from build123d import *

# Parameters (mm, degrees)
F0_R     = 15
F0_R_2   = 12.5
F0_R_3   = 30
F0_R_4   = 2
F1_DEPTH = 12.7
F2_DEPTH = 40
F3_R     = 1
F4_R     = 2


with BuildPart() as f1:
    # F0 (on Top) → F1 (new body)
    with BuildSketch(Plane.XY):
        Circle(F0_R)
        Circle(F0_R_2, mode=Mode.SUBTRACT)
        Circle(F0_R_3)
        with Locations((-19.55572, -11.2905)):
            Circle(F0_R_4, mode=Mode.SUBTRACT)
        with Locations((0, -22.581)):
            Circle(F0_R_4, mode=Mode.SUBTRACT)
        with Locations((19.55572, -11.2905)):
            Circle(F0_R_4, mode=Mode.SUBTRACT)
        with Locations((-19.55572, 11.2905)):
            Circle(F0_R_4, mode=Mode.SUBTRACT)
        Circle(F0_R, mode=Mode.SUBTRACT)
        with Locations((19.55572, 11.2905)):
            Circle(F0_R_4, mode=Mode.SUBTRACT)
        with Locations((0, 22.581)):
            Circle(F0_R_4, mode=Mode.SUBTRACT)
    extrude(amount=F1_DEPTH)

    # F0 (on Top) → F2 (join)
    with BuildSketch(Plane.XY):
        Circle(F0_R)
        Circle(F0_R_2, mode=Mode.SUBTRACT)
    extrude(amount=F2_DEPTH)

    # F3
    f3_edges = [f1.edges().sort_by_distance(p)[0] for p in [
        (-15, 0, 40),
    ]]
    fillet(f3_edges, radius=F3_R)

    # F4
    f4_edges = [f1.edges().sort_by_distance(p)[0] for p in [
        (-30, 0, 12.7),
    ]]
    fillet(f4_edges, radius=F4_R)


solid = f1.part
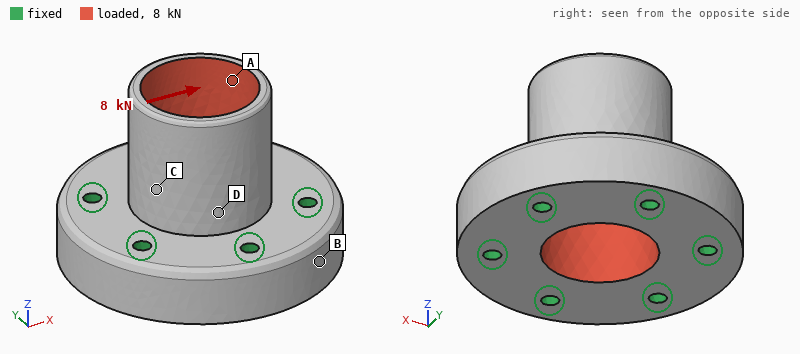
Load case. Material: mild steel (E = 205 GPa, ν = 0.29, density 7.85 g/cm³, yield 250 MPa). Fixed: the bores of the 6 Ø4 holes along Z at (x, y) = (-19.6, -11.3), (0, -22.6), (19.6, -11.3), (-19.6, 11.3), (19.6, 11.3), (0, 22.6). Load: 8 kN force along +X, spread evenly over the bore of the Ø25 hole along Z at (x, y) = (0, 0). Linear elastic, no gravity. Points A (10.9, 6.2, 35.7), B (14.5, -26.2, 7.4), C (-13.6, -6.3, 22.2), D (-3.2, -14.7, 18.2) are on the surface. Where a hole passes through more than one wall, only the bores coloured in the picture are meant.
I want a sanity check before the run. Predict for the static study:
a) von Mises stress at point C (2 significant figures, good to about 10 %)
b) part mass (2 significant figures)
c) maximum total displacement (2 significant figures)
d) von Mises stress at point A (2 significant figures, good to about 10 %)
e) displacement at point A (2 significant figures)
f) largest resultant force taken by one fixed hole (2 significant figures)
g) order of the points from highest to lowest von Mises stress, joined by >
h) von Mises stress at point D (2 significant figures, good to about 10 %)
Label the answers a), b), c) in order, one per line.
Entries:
a) 28 MPa
b) 270 g
c) 17 µm
d) 16 MPa
e) 15 µm
f) 2.2 kN
g) D > C > A > B
h) 53 MPa
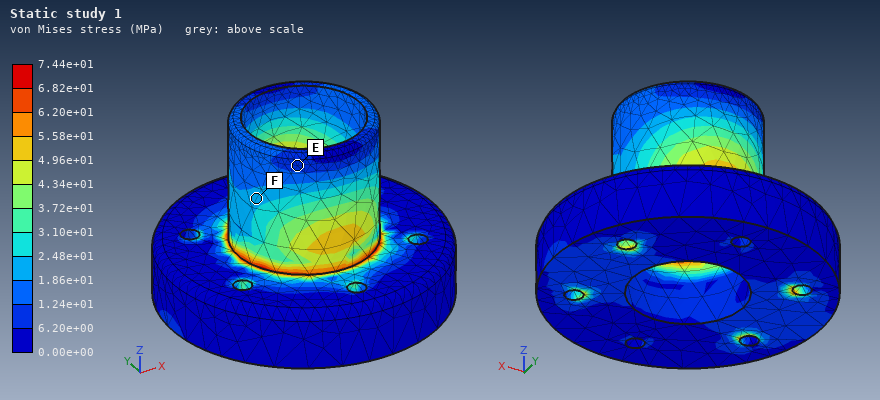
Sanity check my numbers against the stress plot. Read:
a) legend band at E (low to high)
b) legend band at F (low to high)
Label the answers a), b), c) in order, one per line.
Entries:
a) 6.20e+00 to 1.24e+01 MPa
b) 1.86e+01 to 2.48e+01 MPa
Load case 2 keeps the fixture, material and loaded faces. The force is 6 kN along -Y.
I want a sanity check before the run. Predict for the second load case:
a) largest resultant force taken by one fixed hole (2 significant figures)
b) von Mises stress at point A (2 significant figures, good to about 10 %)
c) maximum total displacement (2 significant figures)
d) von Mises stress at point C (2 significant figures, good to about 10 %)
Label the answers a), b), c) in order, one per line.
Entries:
a) 1.8 kN
b) 12 MPa
c) 13 µm
d) 34 MPa
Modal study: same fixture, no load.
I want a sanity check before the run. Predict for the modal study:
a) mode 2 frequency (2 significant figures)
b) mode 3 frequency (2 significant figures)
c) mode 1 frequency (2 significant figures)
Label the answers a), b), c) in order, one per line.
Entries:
a) 12 kHz
b) 15 kHz
c) 12 kHz
